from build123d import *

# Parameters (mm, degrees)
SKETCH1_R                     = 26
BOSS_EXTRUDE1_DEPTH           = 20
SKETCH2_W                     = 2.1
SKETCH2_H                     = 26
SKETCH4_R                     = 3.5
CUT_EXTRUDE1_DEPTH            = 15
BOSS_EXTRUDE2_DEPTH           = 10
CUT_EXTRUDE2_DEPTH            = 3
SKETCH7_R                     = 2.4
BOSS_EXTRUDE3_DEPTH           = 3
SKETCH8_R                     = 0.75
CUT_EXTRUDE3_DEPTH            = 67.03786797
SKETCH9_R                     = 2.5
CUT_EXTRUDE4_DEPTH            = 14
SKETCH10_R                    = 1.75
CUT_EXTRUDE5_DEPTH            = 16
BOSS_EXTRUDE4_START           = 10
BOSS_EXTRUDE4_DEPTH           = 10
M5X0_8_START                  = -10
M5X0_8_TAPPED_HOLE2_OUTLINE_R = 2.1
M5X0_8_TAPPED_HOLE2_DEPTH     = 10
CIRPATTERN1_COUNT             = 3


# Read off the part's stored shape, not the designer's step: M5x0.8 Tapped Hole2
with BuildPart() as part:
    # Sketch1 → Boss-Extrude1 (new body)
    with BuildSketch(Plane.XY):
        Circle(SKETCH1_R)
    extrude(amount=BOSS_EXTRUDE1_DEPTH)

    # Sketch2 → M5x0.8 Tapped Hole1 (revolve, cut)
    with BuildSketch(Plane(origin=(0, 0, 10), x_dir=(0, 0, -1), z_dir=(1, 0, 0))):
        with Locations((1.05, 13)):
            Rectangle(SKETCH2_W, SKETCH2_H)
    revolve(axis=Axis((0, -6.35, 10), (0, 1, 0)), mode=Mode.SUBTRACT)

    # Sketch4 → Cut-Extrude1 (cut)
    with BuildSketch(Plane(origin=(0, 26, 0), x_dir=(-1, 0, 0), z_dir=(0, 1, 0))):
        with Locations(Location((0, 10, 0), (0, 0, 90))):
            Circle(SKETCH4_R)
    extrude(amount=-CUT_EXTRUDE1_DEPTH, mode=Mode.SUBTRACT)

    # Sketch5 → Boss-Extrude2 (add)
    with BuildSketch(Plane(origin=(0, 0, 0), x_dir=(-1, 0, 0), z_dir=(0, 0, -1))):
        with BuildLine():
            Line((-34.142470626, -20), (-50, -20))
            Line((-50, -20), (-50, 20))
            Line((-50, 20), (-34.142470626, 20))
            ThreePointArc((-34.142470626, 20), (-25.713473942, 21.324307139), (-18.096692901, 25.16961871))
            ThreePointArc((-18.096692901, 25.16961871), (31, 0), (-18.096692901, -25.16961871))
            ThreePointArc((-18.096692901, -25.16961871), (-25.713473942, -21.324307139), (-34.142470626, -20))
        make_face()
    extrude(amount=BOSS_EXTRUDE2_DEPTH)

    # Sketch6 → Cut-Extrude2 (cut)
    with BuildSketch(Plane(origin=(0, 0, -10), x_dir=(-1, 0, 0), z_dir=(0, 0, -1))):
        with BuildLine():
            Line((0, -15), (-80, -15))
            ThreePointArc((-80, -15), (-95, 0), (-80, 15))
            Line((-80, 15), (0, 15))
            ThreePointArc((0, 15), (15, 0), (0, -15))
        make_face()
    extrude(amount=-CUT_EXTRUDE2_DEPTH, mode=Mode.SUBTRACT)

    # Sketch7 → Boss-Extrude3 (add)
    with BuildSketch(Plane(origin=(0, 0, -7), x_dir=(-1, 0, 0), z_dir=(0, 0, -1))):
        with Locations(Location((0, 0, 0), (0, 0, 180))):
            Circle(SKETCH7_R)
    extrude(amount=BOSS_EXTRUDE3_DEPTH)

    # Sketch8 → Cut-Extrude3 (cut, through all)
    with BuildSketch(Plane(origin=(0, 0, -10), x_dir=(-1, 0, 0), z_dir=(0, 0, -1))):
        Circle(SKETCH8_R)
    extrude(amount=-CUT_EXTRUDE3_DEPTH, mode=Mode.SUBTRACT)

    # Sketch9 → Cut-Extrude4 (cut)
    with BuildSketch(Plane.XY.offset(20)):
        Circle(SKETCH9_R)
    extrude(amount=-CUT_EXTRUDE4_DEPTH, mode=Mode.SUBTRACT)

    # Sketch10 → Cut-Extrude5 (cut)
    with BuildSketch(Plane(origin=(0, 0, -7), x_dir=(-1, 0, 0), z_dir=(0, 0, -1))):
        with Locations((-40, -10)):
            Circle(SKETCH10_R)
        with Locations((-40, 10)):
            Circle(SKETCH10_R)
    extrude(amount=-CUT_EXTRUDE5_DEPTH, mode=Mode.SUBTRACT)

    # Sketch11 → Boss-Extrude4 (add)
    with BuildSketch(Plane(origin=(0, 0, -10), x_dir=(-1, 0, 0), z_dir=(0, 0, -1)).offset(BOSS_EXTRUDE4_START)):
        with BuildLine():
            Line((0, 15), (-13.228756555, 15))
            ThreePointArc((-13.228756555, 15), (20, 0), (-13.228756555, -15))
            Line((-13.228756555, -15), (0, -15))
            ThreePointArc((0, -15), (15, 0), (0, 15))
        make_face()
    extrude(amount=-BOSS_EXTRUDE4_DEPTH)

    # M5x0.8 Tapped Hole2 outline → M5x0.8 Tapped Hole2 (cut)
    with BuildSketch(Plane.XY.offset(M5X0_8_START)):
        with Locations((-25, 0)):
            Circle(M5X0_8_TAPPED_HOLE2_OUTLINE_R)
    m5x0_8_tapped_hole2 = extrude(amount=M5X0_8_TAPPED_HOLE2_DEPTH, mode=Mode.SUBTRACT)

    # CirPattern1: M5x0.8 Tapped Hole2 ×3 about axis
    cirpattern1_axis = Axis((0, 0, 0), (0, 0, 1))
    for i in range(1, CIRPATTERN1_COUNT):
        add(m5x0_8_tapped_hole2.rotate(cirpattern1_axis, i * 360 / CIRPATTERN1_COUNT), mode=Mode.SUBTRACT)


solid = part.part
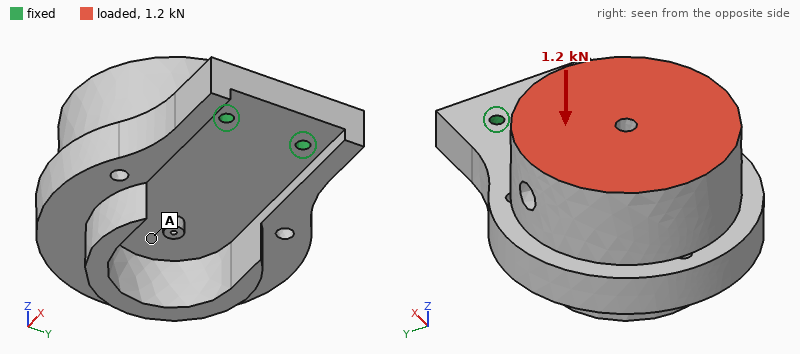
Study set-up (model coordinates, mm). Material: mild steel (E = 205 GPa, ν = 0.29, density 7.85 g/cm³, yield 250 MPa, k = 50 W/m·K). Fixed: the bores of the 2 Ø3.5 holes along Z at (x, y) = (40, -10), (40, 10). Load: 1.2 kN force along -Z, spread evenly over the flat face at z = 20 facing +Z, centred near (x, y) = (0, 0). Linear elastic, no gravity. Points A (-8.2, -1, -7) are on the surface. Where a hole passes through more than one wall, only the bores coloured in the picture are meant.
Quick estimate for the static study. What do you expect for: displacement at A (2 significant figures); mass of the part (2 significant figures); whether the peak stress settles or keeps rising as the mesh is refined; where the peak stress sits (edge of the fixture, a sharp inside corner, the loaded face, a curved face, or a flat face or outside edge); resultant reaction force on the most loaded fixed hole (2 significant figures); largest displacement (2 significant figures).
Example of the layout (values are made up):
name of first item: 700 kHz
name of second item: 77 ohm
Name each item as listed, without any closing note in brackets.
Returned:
displacement at A: 0.10 mm
mass of the part: 610 g
whether the peak stress settles or keeps rising as the mesh is refined: keeps rising
where the peak stress sits: edge of the fixture
resultant reaction force on the most loaded fixed hole: 610 N
largest displacement: 0.16 mm
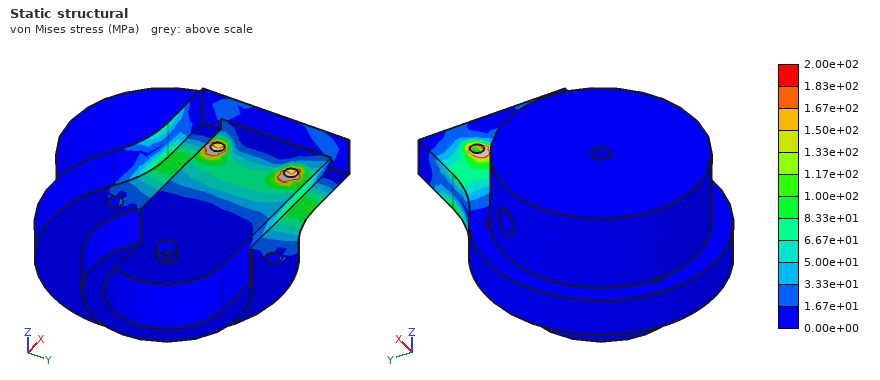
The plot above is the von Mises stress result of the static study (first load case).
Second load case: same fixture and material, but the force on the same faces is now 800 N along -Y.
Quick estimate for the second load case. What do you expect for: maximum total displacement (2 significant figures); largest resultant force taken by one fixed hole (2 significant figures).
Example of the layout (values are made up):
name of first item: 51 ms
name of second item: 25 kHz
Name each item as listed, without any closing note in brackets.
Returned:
maximum total displacement: 18 µm
largest resultant force taken by one fixed hole: 1.7 kN
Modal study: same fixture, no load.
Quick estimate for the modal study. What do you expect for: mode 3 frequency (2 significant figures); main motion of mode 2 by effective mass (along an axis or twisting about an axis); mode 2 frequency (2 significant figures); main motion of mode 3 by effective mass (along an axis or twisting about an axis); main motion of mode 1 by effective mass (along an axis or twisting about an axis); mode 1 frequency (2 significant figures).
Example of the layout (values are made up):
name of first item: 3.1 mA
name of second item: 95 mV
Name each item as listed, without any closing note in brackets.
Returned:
mode 3 frequency: 2900 Hz
main motion of mode 2 by effective mass: along Y
mode 2 frequency: 2200 Hz
main motion of mode 3 by effective mass: along Y
main motion of mode 1 by effective mass: along Z
mode 1 frequency: 710 Hz
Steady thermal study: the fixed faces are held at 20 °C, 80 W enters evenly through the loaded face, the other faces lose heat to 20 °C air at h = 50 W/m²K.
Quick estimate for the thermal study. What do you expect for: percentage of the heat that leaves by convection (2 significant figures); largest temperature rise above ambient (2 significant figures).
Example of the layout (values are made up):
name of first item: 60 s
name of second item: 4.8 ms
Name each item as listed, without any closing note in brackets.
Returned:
percentage of the heat that leaves by convection: 51 %
largest temperature rise above ambient: 83 K
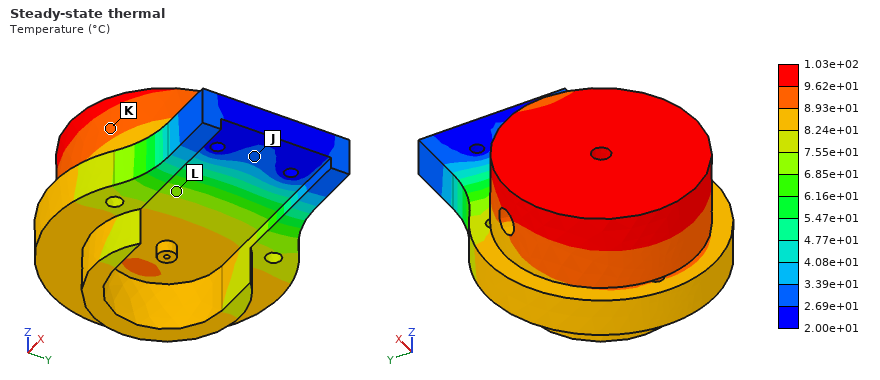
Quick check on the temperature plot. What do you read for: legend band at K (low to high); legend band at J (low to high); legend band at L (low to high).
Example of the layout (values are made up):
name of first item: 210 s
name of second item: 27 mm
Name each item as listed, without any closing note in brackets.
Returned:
legend band at K: 8.93e+01 to 9.62e+01 °C
legend band at J: 2.69e+01 to 3.39e+01 °C
legend band at L: 6.85e+01 to 7.55e+01 °C
